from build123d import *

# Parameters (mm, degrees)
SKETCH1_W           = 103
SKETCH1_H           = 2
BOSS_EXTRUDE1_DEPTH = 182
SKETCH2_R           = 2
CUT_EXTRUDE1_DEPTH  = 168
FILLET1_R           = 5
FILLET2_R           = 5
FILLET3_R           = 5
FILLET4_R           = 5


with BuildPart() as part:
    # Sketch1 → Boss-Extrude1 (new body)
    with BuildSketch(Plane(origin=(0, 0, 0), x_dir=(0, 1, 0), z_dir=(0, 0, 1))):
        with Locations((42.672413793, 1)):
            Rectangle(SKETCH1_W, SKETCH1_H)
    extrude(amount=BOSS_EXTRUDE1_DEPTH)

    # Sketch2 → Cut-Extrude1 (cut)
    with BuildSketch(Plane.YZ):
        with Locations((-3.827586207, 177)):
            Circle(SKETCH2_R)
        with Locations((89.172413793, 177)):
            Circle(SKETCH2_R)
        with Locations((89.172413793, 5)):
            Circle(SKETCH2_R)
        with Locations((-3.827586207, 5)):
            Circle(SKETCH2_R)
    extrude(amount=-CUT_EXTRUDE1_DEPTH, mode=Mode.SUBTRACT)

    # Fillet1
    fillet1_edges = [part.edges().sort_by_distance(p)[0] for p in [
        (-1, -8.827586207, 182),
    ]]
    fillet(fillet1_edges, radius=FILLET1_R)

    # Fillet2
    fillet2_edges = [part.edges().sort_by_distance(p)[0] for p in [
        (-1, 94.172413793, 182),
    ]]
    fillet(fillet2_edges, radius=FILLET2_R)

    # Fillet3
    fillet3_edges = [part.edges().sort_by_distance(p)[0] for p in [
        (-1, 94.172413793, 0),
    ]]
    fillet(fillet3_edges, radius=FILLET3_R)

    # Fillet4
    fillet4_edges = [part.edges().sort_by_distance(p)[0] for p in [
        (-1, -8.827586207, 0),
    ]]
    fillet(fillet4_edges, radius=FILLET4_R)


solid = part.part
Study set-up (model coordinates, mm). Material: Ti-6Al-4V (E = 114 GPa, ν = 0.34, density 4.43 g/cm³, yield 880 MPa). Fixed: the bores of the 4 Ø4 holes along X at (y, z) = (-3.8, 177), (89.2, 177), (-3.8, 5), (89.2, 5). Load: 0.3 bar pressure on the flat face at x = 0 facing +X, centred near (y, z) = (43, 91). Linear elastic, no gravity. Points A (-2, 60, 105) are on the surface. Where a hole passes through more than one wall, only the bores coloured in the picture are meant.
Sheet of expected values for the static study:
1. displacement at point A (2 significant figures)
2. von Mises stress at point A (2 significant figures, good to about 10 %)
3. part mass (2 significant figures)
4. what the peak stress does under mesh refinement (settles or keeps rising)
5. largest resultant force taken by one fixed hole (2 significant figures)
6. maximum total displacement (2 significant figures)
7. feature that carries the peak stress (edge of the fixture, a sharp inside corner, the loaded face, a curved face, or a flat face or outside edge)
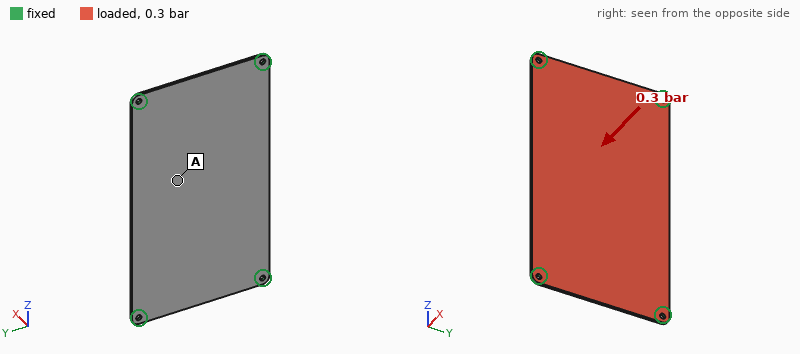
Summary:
1.3 mm
60 MPa
170 g
keeps rising
140 N
1.4 mm
edge of the fixture
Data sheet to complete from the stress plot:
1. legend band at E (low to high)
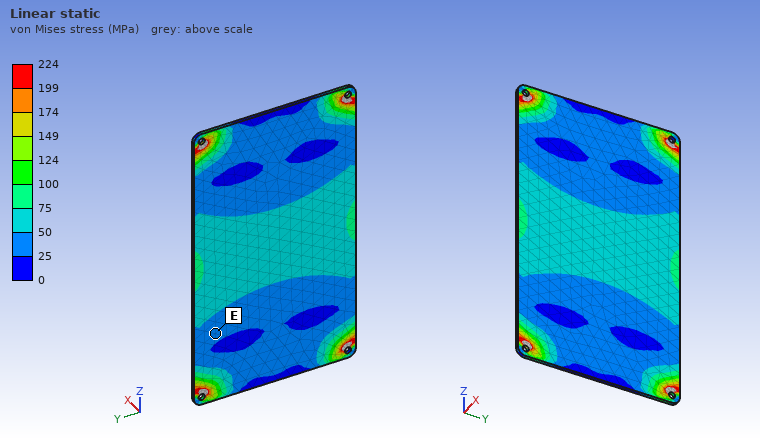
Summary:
25 to 50 MPa
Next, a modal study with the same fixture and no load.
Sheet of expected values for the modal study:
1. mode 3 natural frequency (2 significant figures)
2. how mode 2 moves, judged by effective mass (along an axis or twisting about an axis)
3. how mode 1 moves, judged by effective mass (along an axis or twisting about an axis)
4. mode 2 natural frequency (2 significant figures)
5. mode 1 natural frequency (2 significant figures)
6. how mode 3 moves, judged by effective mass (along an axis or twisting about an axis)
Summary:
780 Hz
twisting about Z
along X
520 Hz
280 Hz
twisting about Y
